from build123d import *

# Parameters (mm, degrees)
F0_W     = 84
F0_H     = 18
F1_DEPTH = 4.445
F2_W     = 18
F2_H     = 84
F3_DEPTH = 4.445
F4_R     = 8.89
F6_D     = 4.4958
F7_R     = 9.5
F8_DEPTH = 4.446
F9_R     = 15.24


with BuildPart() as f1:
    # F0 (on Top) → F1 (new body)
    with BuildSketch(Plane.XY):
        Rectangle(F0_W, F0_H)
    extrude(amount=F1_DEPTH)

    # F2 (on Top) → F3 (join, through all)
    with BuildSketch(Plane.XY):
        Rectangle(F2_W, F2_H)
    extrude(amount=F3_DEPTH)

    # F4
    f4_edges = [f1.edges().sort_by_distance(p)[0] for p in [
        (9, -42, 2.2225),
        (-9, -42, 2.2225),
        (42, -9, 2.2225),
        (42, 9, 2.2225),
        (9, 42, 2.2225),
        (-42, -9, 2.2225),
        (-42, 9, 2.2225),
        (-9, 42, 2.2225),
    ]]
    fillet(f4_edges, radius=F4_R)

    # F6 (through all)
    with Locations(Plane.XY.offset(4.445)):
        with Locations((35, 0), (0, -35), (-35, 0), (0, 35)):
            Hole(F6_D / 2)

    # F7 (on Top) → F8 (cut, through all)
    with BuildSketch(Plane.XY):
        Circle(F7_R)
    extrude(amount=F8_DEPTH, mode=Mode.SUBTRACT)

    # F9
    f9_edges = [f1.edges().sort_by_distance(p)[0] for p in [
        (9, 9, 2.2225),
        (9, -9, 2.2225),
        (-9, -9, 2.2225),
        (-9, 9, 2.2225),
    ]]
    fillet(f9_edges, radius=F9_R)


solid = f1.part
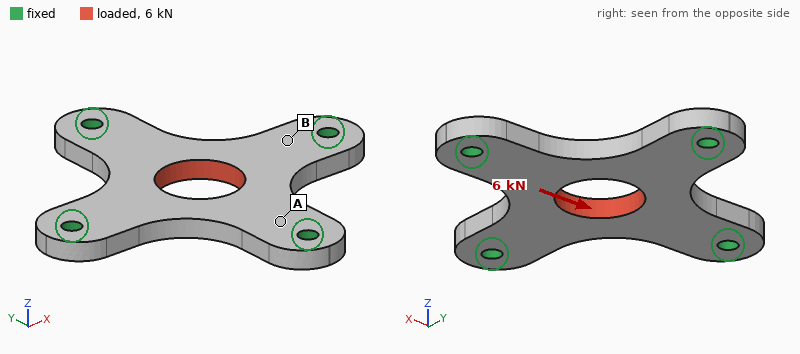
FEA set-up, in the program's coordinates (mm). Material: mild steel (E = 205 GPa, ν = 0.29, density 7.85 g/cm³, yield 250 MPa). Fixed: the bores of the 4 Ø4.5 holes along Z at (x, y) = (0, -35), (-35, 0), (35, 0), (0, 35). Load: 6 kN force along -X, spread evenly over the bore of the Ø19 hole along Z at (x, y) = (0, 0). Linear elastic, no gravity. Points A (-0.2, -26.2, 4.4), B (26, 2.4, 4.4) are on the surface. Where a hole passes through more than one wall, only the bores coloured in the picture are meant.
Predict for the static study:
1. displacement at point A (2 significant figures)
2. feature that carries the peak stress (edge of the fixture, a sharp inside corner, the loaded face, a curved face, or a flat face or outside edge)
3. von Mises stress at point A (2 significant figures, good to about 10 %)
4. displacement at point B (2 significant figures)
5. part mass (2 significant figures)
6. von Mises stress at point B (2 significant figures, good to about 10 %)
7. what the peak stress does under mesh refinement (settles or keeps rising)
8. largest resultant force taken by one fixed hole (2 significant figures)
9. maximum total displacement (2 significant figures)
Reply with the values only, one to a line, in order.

1.9 µm
edge of the fixture
12 MPa
1.8 µm
84 g
38 MPa
keeps rising
2.6 kN
5.9 µm
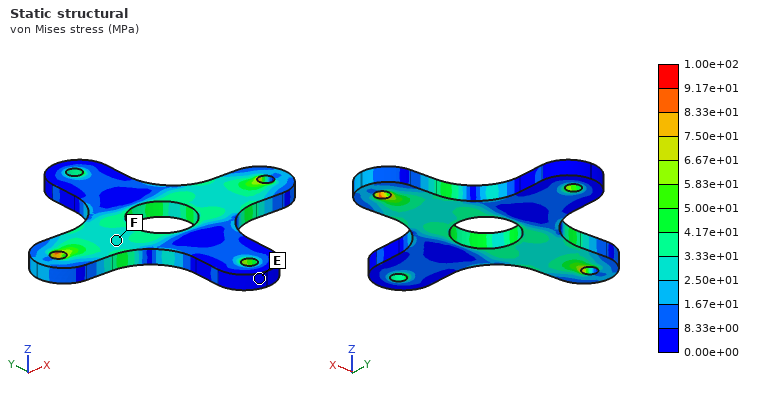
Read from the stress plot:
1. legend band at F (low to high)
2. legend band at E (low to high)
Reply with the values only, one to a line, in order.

2.50e+01 to 3.33e+01 MPa
0.00e+00 to 8.33e+00 MPa
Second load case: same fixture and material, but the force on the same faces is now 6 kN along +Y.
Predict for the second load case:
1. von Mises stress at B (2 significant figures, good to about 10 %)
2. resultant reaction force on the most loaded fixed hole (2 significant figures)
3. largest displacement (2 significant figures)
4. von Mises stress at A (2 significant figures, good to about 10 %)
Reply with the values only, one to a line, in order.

11 MPa
2.6 kN
5.9 µm
40 MPa
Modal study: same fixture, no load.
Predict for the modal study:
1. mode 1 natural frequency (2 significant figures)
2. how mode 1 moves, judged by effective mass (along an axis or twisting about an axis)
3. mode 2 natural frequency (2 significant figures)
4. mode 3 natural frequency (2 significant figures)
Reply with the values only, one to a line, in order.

6600 Hz
along Z
12 kHz
12 kHz
